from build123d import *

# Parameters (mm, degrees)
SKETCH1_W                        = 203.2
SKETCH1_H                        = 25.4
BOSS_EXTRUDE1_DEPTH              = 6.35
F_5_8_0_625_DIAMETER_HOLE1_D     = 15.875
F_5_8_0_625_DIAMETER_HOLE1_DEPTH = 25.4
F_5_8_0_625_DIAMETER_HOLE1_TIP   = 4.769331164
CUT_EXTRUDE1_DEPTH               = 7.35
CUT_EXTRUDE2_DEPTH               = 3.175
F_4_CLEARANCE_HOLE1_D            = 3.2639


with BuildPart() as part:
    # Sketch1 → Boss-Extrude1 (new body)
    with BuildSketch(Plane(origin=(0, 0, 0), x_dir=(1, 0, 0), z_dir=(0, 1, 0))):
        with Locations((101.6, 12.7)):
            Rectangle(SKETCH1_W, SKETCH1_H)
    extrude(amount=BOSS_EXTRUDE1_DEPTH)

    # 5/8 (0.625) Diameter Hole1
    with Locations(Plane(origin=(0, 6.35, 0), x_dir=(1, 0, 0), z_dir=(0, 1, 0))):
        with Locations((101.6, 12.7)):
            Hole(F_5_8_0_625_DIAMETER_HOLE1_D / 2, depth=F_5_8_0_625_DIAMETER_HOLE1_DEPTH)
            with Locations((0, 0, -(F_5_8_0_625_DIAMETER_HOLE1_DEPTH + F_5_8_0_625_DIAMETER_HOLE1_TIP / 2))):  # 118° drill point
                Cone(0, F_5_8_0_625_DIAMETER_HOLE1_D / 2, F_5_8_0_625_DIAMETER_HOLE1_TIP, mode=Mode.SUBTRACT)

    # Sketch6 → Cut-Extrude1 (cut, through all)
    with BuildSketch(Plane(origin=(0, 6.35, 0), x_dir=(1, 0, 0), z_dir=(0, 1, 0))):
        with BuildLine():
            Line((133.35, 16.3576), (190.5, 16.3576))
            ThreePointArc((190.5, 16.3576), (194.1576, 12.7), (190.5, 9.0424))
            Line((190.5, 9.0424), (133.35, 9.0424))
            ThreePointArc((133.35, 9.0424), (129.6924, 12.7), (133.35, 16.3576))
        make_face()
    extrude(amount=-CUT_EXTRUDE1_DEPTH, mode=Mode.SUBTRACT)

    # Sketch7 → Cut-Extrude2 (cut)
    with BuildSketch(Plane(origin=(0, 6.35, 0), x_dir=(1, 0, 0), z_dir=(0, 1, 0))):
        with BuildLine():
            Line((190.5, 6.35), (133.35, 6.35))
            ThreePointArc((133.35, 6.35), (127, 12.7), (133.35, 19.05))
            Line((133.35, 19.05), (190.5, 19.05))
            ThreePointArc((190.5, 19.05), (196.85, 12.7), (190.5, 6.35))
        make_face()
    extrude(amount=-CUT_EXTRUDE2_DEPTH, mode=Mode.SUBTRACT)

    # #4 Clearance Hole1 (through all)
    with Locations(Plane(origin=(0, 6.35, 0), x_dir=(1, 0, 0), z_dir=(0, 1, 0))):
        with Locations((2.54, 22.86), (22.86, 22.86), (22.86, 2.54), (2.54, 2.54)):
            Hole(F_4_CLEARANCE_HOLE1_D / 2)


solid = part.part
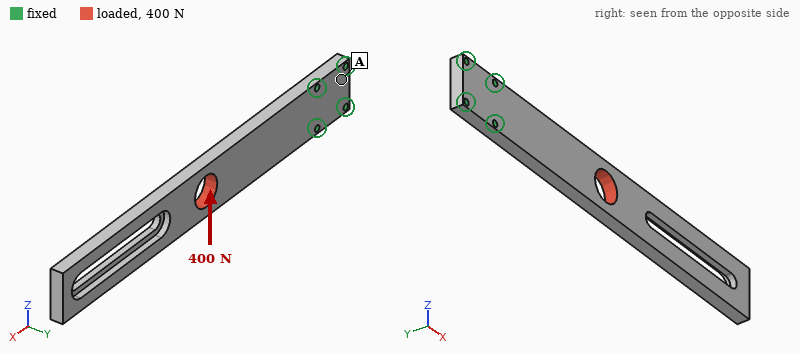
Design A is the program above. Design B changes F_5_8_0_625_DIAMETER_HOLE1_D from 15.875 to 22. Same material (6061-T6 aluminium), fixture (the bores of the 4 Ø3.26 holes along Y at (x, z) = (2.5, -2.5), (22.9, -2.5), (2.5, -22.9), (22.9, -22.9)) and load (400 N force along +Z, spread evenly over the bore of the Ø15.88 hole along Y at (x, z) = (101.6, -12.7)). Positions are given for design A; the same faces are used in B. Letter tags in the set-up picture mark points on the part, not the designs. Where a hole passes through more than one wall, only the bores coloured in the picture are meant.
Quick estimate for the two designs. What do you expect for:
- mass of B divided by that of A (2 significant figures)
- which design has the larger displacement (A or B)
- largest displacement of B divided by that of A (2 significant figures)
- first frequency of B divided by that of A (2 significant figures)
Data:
0.96
B
1.2
0.91
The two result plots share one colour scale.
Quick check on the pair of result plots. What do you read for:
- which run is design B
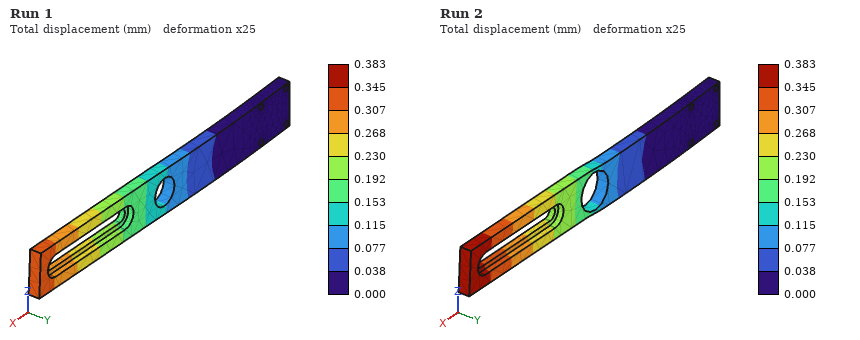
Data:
Run 2
